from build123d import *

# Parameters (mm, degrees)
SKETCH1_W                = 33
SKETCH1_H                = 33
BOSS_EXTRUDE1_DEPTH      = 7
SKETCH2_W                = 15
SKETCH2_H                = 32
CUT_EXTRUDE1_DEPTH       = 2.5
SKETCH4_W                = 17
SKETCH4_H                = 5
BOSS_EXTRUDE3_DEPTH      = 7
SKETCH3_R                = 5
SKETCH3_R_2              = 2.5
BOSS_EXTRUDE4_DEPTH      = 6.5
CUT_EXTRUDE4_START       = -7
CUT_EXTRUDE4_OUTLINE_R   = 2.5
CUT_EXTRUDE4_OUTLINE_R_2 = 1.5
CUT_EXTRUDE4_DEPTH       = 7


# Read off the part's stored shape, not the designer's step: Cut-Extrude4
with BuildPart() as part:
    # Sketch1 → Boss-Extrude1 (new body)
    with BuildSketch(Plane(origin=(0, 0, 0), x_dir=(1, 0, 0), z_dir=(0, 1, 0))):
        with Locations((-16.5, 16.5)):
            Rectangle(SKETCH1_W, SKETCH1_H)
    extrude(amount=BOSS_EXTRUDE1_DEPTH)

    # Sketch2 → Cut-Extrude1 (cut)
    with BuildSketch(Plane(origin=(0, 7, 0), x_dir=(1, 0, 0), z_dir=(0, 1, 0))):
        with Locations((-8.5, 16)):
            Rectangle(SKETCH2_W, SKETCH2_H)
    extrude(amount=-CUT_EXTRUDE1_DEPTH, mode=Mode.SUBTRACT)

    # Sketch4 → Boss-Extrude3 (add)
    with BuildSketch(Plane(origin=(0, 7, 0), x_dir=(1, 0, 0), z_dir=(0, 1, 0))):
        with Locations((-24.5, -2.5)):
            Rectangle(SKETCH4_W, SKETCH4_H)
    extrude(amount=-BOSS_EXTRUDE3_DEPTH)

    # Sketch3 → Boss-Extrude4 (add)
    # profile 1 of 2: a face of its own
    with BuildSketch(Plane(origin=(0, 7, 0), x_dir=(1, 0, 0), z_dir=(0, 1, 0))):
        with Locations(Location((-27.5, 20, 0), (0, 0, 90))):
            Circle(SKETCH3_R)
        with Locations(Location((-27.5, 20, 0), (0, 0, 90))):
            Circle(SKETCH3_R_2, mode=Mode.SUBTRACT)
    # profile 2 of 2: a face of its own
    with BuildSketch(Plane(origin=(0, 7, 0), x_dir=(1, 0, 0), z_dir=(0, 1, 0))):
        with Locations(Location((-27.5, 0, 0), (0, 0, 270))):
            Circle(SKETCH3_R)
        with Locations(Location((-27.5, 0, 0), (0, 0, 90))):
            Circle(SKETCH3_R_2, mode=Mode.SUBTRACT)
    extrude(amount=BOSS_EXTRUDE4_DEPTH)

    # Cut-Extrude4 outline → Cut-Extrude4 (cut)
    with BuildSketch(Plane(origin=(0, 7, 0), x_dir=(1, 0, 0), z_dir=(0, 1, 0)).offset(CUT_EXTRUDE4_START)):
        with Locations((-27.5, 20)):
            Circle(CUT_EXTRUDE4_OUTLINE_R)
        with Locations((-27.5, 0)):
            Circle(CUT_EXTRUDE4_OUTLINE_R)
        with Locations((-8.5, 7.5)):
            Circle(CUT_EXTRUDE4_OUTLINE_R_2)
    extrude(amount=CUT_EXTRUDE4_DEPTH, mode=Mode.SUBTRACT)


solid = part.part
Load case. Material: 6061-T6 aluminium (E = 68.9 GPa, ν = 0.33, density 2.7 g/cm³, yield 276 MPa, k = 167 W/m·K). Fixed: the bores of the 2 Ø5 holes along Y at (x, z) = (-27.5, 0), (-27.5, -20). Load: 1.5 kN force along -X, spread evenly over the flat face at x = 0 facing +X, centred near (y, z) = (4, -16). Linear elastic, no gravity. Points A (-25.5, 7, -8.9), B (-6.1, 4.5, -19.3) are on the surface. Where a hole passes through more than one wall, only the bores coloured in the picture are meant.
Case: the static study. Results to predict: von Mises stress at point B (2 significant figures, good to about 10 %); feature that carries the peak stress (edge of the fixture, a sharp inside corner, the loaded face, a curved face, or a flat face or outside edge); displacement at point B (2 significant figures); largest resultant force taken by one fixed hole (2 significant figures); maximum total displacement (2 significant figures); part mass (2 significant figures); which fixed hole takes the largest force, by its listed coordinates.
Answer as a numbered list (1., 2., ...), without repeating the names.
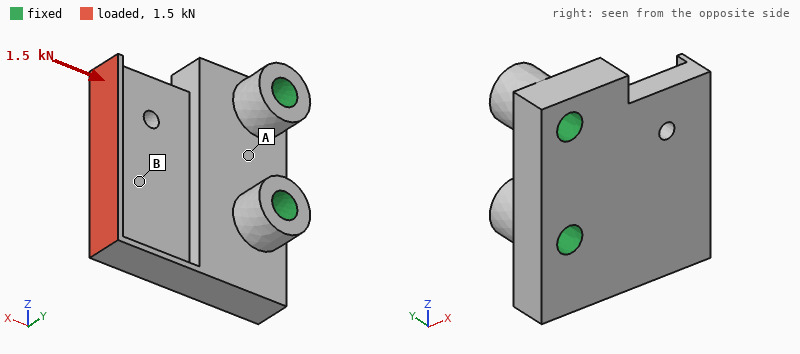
1. 25 MPa
2. the loaded face
3. 8.3 µm
4. 1.1 kN
5. 28 µm
6. 20 g
7. (-27.5, -20)
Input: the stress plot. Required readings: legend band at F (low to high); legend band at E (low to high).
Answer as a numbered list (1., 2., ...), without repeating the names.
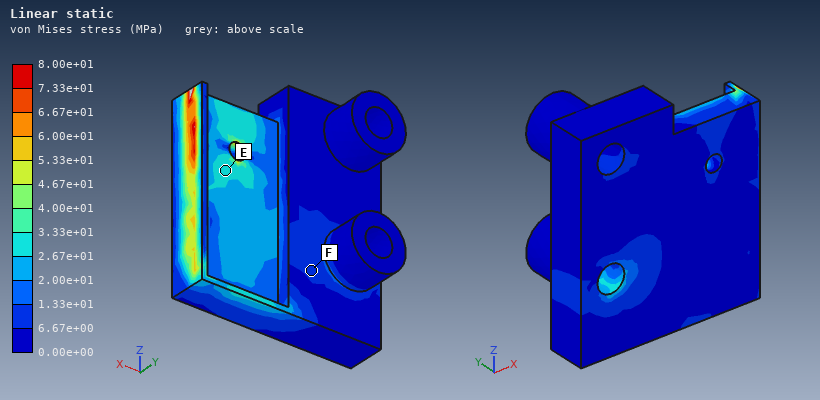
1. 6.67e+00 to 1.33e+01 MPa
2. 2.67e+01 to 3.33e+01 MPa
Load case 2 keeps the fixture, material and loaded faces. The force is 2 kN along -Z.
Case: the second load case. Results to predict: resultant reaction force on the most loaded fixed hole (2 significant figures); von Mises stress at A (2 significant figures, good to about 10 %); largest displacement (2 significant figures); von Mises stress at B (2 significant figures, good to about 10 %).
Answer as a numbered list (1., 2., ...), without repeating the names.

1. 2.5 kN
2. 15 MPa
3. 54 µm
4. 50 MPa
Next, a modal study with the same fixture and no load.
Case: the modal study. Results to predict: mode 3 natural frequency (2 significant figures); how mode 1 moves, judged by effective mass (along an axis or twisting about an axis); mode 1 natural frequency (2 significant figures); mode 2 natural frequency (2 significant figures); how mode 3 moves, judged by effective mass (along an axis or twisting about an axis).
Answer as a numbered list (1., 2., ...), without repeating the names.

1. 20 kHz
2. along Y
3. 7900 Hz
4. 12 kHz
5. along Z
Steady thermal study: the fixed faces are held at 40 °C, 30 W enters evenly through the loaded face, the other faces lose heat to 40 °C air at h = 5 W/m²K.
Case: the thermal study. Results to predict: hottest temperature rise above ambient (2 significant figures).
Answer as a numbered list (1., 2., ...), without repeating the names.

1. 32 K
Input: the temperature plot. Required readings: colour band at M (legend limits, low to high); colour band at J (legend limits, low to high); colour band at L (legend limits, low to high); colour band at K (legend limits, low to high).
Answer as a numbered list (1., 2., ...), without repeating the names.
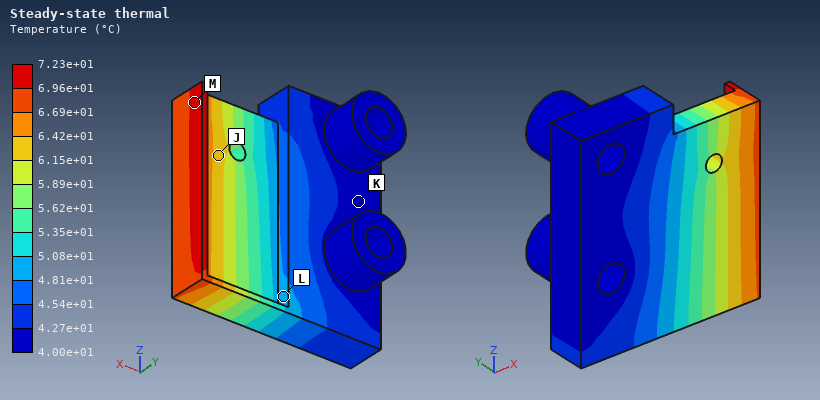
1. 6.96e+01 to 7.23e+01 °C
2. 6.15e+01 to 6.42e+01 °C
3. 4.81e+01 to 5.08e+01 °C
4. 4.00e+01 to 4.27e+01 °C
